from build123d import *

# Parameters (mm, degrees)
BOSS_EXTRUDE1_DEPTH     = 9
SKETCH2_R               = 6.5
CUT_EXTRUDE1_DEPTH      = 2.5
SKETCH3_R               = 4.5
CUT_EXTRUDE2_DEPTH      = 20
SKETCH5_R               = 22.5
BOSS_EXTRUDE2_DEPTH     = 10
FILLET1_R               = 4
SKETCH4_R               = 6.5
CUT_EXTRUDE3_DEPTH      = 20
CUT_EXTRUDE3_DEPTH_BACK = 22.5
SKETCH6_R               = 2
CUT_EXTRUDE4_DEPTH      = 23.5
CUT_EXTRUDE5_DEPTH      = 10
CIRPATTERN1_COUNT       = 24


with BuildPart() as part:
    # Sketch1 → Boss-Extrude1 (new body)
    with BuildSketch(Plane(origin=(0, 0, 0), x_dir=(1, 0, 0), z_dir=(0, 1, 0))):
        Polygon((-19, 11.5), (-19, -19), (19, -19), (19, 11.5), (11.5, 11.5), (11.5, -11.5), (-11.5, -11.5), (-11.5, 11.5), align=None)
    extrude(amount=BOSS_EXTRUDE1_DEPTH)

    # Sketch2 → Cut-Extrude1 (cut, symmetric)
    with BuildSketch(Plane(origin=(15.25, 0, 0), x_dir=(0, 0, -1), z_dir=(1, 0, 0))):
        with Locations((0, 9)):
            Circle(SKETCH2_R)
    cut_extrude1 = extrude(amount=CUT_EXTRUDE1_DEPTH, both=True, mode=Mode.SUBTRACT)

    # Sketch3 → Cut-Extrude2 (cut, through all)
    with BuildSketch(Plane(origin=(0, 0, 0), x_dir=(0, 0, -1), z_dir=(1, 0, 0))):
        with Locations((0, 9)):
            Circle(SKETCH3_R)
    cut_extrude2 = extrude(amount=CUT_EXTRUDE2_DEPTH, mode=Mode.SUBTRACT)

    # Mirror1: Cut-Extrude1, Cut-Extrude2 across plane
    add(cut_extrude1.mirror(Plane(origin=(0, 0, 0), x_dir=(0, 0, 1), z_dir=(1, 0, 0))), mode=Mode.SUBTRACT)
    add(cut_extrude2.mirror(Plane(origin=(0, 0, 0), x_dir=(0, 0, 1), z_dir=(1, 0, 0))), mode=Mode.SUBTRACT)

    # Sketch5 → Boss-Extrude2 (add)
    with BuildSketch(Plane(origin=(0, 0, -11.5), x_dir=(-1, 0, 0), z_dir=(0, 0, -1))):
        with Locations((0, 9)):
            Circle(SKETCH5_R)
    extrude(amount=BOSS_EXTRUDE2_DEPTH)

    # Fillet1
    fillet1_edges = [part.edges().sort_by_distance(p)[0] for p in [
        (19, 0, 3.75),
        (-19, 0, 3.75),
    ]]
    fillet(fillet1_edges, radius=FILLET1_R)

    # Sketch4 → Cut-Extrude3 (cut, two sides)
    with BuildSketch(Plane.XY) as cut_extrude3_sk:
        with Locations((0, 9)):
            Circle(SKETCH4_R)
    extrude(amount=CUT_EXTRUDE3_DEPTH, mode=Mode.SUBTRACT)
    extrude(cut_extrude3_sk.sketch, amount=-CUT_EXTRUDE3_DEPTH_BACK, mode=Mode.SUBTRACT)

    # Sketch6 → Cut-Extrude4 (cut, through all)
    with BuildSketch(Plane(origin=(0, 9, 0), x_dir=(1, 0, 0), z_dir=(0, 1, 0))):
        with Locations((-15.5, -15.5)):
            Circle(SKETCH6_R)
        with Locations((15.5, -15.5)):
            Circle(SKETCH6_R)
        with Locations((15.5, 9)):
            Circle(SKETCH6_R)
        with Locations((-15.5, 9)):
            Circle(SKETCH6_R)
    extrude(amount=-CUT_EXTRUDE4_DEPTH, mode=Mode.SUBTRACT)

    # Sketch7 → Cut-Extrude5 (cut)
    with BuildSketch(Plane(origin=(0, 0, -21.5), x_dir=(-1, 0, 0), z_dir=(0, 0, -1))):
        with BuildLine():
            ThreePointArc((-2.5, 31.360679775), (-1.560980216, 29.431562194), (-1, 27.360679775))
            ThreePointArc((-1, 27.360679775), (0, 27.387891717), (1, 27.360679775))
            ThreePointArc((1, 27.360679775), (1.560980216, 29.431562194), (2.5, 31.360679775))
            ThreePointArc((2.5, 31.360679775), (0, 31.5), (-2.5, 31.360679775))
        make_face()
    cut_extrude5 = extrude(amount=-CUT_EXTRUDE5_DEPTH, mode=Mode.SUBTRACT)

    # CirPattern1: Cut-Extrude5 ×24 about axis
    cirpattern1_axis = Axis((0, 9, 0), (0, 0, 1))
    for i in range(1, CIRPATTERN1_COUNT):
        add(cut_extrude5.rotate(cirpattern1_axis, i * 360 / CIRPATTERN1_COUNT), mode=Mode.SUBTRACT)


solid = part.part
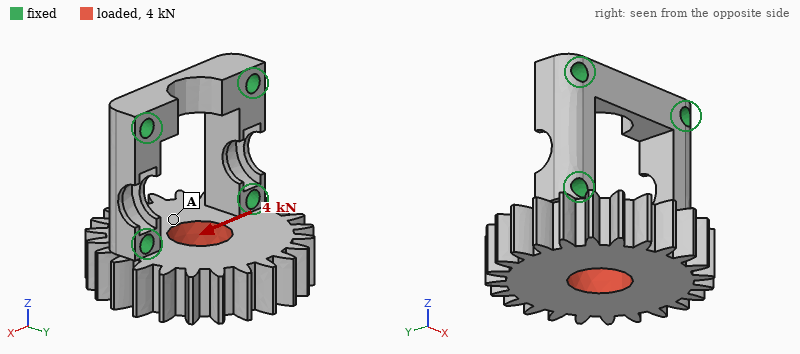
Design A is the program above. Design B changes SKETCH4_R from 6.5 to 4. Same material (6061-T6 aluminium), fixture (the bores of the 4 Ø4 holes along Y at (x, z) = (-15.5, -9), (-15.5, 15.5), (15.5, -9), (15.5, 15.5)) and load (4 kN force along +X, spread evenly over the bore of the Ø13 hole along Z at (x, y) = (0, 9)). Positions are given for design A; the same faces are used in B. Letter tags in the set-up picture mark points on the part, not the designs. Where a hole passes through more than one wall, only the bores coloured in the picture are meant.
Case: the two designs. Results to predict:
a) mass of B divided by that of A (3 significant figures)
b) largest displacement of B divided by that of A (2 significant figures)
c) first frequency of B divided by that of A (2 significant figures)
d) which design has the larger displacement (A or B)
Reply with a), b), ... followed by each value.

a) 1.08
b) 0.83
c) 1.00
d) A
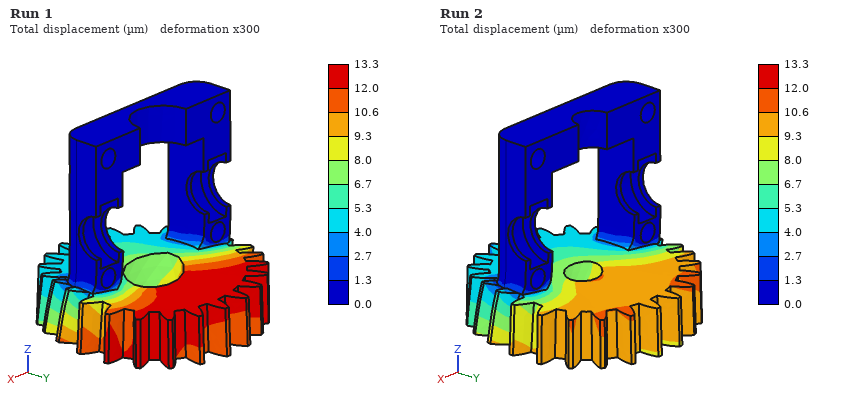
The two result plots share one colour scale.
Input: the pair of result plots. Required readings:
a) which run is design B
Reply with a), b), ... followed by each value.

a) Run 2
